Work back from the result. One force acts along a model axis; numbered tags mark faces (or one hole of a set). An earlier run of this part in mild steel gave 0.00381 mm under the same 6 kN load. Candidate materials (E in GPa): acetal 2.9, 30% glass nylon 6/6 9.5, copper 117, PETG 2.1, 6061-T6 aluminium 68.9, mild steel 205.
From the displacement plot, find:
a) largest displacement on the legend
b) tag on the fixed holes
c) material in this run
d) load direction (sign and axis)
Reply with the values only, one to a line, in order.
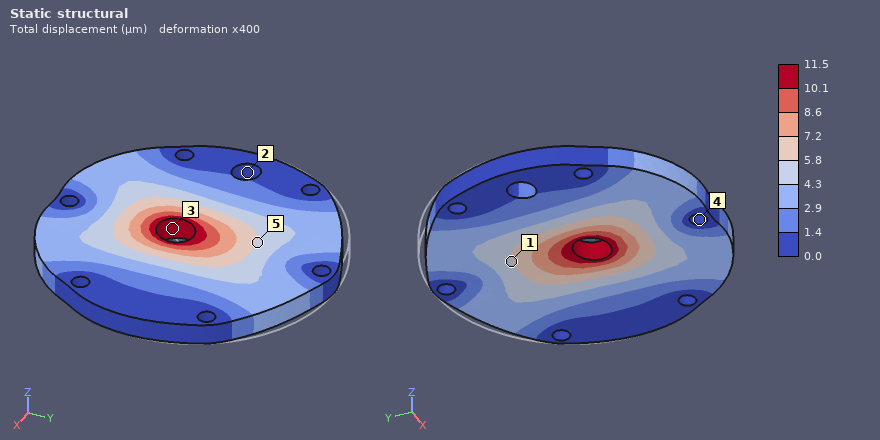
11.5 µm
4
6061-T6 aluminium
-Y
